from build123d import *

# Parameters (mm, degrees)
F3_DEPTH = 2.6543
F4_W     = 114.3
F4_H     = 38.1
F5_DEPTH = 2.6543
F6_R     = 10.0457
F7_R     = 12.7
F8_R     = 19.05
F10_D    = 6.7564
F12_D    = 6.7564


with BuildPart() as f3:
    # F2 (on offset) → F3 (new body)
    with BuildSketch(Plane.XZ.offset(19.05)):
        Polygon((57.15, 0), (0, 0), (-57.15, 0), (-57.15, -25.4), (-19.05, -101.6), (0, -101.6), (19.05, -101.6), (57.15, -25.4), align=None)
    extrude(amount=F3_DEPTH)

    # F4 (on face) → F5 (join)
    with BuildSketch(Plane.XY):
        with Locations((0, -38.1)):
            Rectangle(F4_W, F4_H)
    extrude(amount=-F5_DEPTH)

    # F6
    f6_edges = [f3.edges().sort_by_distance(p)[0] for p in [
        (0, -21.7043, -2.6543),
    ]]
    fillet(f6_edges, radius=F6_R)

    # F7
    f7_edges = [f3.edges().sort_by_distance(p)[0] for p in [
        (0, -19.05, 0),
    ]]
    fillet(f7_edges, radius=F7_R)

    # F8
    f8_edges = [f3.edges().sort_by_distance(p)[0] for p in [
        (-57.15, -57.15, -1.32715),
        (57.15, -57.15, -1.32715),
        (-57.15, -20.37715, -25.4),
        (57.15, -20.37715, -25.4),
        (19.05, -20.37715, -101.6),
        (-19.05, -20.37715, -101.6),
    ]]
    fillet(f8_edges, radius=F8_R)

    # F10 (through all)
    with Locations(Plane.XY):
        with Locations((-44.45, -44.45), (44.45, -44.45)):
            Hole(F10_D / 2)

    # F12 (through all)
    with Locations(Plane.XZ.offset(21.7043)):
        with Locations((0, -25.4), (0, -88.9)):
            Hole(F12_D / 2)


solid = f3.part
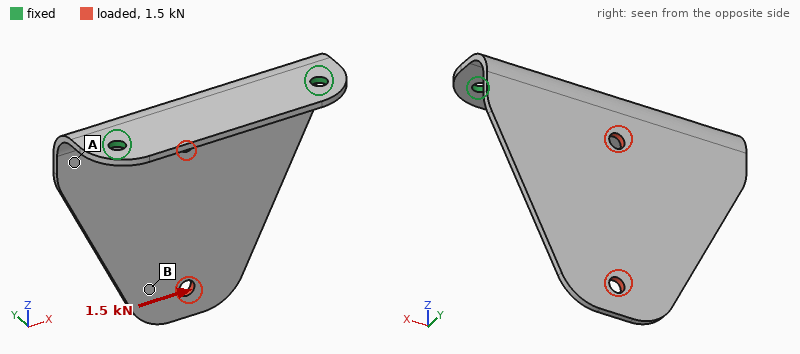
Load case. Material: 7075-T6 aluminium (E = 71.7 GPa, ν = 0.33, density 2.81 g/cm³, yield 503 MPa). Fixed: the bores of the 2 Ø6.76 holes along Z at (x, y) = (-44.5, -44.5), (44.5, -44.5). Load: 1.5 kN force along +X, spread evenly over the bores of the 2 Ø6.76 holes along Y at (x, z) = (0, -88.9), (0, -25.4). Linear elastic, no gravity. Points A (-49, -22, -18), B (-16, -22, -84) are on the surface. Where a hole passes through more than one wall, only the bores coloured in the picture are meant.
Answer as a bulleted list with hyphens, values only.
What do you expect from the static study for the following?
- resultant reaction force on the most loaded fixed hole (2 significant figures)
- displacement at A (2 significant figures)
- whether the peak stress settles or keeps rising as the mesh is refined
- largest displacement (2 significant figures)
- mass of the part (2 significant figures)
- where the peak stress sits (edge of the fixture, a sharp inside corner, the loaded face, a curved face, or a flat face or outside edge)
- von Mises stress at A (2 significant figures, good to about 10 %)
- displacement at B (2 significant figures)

- 1.3 kN
- 0.81 mm
- keeps rising
- 1.4 mm
- 88 g
- edge of the fixture
- 100 MPa
- 1.2 mm
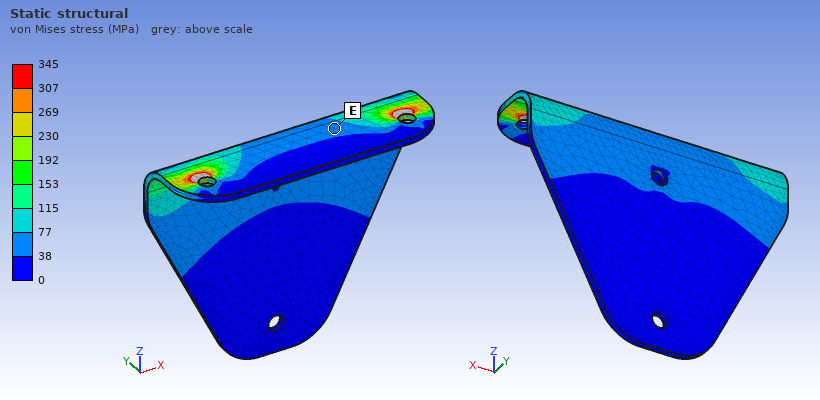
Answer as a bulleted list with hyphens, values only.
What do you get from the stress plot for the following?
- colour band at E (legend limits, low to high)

- 38 to 77 MPa
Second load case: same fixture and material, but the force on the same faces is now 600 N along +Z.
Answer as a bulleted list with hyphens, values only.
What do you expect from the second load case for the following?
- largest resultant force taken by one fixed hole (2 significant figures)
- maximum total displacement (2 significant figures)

- 300 N
- 1.7 mm
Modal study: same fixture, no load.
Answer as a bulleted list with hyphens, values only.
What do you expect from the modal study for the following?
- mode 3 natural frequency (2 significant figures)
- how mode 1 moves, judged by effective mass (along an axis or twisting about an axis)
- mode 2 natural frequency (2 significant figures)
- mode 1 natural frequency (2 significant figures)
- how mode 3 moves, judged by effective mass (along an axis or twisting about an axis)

- 970 Hz
- along Y
- 700 Hz
- 220 Hz
- along Z
